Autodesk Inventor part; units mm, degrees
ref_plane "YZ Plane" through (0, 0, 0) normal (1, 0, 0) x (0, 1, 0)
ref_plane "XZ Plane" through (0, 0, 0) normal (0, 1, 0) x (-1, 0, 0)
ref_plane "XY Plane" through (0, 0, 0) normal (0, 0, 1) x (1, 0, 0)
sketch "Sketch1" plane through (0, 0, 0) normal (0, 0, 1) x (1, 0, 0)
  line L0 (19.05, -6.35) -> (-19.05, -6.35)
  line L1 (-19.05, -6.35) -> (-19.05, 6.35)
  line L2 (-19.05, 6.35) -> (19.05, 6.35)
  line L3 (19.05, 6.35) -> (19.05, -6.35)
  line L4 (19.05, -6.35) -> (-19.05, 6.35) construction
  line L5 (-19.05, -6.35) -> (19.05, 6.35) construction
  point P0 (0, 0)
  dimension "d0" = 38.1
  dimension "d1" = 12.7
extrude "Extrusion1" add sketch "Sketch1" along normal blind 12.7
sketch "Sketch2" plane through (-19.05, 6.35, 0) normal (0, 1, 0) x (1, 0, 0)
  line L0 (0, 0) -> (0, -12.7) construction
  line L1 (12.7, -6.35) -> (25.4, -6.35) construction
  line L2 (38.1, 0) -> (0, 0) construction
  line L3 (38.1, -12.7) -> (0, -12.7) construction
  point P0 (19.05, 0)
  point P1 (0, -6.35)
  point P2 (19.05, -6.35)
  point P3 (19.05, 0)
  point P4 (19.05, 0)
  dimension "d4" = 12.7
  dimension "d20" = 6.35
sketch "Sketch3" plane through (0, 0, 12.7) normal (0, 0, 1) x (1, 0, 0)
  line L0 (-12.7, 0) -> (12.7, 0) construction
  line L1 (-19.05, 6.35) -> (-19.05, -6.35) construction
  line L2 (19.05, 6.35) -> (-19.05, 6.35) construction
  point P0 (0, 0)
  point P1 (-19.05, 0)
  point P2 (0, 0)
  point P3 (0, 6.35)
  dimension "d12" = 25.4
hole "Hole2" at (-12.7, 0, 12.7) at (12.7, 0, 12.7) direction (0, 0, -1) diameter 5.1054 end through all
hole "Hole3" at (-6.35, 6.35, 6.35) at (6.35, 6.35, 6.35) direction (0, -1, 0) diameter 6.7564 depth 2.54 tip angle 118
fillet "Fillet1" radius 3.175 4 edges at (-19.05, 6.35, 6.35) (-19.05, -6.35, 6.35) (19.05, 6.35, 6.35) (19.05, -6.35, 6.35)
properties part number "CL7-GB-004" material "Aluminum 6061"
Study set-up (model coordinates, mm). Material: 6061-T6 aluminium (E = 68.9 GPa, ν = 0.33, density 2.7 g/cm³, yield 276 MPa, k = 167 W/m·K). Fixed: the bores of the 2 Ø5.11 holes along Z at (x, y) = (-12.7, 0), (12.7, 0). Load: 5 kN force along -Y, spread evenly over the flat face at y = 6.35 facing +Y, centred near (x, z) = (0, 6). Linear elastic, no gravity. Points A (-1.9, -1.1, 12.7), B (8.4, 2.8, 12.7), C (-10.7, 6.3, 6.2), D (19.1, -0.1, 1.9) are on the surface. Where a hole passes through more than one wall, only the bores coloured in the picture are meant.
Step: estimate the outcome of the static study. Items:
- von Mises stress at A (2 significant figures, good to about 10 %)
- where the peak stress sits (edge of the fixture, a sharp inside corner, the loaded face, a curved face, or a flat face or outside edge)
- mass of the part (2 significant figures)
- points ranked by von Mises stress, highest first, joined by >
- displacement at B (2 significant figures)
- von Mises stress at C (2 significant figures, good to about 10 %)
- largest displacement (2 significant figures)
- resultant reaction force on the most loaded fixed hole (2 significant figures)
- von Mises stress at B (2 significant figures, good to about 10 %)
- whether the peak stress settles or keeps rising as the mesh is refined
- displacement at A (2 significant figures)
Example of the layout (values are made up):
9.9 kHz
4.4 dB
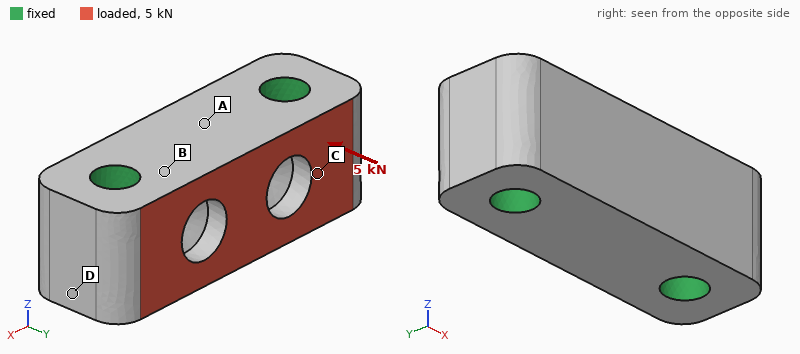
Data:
8.0 MPa
edge of the fixture
14 g
B > C > A > D
2.1 µm
18 MPa
5.3 µm
2.5 kN
23 MPa
keeps rising
4.2 µm
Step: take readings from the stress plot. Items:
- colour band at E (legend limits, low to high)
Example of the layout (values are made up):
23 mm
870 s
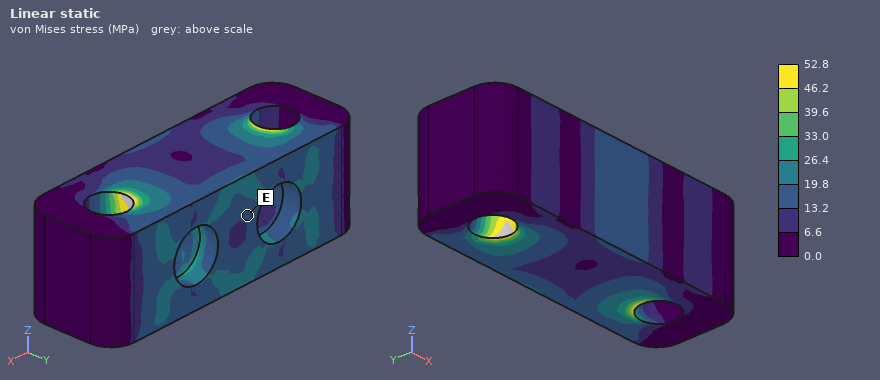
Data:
13.2 to 19.8 MPa
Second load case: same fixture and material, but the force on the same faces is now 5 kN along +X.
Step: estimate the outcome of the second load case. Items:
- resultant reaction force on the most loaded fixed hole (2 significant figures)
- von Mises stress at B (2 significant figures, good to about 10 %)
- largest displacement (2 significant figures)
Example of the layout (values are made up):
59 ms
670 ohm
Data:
2.6 kN
29 MPa
5.1 µm
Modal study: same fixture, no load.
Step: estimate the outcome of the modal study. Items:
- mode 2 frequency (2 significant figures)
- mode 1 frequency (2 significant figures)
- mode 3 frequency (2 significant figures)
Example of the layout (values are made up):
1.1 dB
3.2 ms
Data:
51 kHz
50 kHz
59 kHz
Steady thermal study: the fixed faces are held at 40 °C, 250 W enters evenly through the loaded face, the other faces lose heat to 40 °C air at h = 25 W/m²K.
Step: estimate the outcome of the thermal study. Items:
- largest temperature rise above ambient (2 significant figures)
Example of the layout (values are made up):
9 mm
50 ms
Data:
41 K
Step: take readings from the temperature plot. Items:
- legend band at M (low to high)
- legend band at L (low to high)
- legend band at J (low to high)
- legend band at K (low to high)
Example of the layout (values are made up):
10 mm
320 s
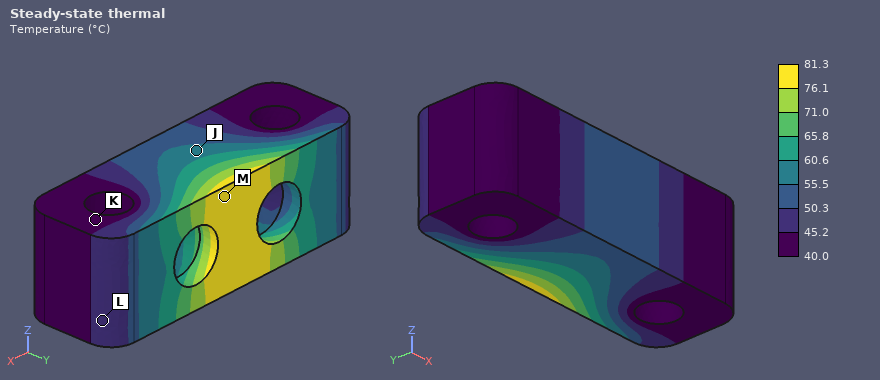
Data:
76.1 to 81.3 °C
45.2 to 50.3 °C
55.5 to 60.6 °C
40.0 to 45.2 °C
